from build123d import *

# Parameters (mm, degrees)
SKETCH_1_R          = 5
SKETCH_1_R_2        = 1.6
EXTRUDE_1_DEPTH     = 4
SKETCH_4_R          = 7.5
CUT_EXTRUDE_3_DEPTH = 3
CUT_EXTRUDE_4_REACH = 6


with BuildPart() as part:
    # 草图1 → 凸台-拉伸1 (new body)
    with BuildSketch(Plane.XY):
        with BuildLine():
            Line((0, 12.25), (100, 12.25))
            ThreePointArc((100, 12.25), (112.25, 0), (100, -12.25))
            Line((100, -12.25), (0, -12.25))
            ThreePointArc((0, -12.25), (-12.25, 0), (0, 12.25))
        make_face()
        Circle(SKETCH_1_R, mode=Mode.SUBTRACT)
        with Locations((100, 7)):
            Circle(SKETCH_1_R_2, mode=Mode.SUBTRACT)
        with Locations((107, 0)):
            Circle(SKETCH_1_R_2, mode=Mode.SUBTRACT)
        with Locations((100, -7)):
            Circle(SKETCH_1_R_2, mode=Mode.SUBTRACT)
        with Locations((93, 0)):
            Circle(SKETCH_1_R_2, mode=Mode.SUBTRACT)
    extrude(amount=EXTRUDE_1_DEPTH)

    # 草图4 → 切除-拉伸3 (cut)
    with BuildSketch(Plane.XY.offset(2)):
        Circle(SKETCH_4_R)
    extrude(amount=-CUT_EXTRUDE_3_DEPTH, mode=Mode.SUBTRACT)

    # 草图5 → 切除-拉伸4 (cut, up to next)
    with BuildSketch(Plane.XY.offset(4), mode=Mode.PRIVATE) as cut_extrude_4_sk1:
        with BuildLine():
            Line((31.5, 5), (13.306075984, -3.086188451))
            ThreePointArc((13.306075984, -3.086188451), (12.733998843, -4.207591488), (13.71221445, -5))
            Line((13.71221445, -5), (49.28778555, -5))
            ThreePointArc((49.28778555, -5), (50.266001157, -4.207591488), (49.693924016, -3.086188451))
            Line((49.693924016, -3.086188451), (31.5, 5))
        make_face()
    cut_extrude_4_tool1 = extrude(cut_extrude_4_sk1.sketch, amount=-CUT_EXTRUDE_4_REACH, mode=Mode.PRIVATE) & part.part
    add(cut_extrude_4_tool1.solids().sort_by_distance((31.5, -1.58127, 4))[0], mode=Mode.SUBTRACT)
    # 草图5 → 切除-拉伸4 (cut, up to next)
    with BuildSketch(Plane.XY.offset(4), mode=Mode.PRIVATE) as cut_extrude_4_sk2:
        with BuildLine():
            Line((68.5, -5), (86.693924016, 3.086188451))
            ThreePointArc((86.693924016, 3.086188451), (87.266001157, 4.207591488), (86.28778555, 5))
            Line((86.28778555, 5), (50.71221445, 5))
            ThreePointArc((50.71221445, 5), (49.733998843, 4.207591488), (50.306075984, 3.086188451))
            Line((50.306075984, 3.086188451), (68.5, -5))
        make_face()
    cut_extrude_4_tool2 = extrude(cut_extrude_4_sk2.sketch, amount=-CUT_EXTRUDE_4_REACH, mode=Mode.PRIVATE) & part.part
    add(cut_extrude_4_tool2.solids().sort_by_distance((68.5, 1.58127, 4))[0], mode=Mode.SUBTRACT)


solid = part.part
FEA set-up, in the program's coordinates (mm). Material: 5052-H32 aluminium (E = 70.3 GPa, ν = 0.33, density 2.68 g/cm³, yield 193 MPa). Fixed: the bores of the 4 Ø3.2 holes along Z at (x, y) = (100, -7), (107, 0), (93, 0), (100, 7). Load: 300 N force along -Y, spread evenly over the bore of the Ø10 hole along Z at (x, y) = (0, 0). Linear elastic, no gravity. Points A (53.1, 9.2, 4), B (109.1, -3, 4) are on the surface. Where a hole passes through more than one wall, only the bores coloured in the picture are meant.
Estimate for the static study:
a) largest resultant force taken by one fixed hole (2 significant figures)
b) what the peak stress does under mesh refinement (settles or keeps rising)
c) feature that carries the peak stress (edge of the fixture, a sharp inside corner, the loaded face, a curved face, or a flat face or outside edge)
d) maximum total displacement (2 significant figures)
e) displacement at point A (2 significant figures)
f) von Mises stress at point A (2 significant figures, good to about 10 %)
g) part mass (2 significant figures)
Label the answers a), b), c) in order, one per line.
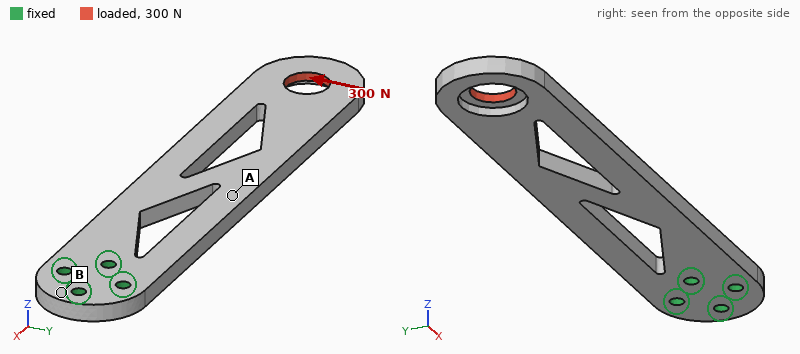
a) 1.4 kN
b) keeps rising
c) edge of the fixture
d) 0.43 mm
e) 0.12 mm
f) 40 MPa
g) 25 g
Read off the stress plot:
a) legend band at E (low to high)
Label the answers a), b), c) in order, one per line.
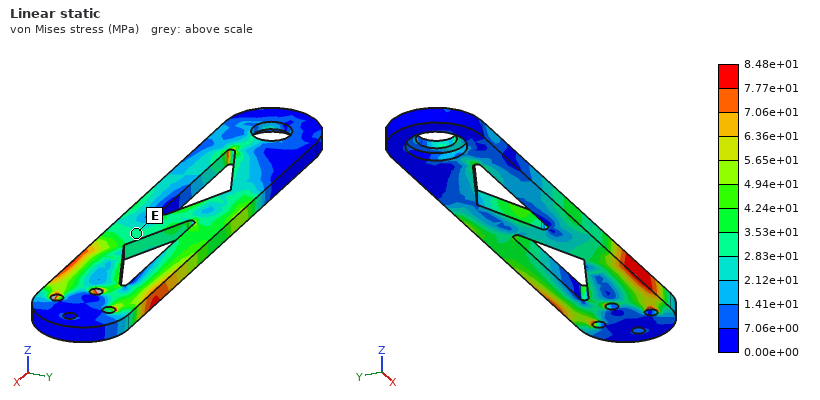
a) 2.83e+01 to 3.53e+01 MPa
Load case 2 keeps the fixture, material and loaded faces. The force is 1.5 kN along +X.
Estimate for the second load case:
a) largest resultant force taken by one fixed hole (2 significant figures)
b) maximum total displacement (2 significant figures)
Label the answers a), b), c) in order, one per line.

a) 510 N
b) 1.2 mm
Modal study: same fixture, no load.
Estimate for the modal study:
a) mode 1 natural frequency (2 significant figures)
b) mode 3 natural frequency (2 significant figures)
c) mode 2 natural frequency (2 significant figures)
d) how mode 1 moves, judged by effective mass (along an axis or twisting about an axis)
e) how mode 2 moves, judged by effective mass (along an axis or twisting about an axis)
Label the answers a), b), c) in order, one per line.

a) 310 Hz
b) 1900 Hz
c) 1600 Hz
d) along Z
e) along Y
